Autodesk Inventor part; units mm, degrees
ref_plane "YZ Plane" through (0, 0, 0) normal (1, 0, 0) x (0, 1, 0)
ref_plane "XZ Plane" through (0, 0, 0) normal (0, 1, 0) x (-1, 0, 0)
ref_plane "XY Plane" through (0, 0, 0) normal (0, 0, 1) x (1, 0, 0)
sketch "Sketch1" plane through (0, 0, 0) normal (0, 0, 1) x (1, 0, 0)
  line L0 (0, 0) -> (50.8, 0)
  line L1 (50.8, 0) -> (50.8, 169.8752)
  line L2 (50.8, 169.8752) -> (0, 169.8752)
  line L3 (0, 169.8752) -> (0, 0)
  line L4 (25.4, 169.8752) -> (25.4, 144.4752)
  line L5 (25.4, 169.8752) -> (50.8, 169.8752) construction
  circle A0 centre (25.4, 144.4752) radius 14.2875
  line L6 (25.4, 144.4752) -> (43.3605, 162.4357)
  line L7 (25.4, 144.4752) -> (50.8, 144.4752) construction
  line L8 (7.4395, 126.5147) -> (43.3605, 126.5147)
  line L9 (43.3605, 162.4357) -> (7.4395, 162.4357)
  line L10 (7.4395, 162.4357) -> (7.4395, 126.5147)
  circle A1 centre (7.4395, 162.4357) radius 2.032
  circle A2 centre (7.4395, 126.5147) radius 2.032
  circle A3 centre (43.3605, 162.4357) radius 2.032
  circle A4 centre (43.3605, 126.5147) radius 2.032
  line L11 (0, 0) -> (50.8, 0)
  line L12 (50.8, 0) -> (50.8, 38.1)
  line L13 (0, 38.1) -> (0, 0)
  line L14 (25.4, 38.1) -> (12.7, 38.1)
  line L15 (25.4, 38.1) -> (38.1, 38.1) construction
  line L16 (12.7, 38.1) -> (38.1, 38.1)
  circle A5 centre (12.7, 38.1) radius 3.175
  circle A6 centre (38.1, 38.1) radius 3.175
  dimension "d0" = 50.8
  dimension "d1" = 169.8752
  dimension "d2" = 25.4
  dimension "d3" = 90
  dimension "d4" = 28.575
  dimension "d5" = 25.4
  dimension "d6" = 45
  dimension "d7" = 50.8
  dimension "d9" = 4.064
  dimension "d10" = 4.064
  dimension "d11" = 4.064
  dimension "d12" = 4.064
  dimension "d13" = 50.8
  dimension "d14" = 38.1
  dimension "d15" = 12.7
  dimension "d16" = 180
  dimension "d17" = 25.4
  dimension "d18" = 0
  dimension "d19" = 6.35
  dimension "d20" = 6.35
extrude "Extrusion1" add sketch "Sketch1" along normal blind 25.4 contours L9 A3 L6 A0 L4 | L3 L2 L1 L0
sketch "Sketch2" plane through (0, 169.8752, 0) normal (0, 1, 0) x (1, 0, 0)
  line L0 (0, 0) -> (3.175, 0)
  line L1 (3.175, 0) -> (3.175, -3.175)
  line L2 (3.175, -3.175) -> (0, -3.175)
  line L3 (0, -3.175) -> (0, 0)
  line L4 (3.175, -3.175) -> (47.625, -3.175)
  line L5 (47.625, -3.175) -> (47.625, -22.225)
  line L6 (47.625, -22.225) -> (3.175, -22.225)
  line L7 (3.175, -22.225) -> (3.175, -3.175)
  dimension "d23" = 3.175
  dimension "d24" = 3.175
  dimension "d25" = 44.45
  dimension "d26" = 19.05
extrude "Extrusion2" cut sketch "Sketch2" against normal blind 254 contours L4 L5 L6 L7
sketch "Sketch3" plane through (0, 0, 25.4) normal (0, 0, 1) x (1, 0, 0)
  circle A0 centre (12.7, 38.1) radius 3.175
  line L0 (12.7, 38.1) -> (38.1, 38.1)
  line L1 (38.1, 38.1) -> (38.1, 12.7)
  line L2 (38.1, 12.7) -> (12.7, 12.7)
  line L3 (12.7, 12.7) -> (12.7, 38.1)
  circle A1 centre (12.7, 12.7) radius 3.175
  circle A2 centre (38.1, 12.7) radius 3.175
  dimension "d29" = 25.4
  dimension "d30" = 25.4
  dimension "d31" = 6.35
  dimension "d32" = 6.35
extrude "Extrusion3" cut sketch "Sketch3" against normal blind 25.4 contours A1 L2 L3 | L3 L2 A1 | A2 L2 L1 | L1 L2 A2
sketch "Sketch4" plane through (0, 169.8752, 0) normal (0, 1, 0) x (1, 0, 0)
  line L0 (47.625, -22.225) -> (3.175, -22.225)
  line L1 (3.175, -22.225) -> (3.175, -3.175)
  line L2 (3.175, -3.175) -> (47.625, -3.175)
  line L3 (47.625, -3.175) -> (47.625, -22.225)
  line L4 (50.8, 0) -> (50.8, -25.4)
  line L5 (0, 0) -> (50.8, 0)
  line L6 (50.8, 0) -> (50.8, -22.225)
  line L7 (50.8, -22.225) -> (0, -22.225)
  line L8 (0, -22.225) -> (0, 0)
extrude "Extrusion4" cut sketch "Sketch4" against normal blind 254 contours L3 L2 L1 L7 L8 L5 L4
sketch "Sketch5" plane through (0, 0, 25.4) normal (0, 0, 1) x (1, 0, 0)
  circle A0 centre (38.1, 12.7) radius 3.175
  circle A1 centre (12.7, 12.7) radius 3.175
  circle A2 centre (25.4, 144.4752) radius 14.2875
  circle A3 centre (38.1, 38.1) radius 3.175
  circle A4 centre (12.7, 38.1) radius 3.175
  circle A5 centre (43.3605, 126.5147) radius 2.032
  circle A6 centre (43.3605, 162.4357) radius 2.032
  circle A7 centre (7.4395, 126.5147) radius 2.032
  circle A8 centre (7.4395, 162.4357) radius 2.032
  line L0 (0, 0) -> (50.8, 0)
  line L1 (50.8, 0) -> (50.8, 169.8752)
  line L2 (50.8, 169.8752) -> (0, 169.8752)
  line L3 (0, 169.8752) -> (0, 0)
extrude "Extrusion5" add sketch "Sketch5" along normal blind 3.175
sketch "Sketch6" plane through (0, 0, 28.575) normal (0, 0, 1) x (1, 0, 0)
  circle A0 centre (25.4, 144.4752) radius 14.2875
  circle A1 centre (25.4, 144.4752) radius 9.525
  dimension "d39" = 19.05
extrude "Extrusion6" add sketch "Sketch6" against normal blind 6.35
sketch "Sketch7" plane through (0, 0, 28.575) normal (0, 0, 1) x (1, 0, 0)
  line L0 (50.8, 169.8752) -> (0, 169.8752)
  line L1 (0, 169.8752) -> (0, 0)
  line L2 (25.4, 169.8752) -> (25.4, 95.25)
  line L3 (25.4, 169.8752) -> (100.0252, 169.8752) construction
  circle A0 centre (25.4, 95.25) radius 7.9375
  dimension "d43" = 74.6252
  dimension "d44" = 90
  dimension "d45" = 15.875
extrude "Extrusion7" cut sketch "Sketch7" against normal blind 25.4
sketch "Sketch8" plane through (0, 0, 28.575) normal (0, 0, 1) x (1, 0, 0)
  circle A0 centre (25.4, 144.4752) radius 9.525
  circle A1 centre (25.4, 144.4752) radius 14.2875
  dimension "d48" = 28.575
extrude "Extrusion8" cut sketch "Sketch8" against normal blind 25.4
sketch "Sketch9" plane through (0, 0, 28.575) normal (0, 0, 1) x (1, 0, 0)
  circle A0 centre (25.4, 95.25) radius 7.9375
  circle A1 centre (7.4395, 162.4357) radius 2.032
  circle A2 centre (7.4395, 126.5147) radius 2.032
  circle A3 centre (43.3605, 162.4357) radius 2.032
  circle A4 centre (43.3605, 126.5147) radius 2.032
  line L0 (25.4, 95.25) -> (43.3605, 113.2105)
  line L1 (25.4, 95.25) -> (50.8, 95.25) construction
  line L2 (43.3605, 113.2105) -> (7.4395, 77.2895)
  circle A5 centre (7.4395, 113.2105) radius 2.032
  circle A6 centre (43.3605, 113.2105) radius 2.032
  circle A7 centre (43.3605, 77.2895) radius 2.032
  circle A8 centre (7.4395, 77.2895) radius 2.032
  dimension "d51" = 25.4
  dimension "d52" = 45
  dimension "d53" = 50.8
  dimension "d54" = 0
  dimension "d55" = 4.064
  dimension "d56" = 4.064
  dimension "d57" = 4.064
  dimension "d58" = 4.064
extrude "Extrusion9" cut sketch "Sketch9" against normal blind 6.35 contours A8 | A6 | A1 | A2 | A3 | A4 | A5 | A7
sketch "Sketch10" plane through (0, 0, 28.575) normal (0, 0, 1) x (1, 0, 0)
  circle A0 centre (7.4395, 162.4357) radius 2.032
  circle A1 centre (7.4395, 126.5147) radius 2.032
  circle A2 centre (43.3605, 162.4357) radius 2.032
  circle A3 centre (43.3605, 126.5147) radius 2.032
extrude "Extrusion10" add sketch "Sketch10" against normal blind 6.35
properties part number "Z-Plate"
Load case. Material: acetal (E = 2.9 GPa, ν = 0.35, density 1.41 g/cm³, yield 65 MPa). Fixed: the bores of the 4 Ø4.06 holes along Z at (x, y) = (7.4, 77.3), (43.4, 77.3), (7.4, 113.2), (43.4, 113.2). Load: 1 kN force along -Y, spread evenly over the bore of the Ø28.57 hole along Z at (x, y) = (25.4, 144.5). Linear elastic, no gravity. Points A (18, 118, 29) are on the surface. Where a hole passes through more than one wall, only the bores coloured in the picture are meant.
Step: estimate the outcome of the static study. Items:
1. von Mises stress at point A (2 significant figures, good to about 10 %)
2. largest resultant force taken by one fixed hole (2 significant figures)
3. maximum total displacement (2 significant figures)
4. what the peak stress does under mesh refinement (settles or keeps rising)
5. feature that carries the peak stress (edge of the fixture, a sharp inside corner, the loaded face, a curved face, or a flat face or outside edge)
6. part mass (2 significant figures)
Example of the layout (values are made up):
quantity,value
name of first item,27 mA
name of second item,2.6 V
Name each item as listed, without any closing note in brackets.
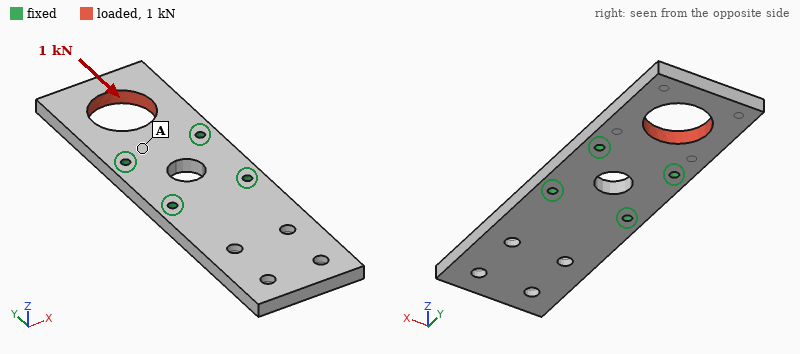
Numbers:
quantity,value
von Mises stress at point A,1.2 MPa
largest resultant force taken by one fixed hole,450 N
maximum total displacement,0.12 mm
what the peak stress does under mesh refinement,keeps rising
feature that carries the peak stress,edge of the fixture
part mass,68 g
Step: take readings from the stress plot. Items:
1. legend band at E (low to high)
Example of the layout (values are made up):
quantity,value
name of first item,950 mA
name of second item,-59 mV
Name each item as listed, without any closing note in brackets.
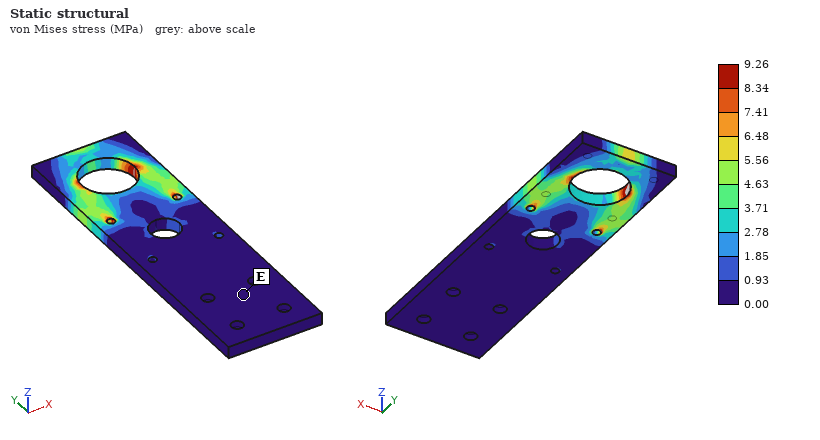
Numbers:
quantity,value
legend band at E,0.00 to 0.93 MPa
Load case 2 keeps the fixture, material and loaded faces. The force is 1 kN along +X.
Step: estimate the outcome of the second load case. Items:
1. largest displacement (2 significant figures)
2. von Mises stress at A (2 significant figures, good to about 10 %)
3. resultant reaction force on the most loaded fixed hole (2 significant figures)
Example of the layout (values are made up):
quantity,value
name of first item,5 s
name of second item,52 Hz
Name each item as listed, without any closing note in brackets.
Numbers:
quantity,value
largest displacement,0.57 mm
von Mises stress at A,8.3 MPa
resultant reaction force on the most loaded fixed hole,890 N
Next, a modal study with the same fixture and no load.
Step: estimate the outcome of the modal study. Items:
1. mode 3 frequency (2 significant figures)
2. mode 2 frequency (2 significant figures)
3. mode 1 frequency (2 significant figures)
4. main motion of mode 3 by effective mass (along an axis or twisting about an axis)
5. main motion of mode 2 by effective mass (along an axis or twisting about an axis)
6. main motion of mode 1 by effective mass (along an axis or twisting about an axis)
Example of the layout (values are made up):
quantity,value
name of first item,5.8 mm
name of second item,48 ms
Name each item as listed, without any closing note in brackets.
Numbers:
quantity,value
mode 3 frequency,800 Hz
mode 2 frequency,420 Hz
mode 1 frequency,240 Hz
main motion of mode 3 by effective mass,twisting about Y
main motion of mode 2 by effective mass,along Z
main motion of mode 1 by effective mass,along Z
